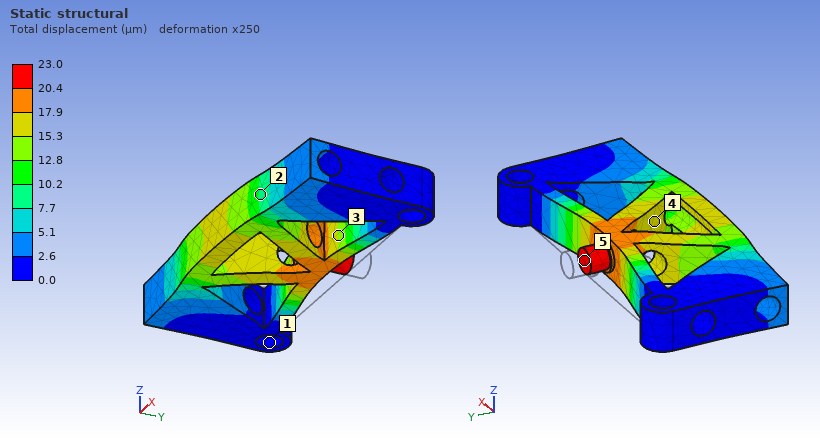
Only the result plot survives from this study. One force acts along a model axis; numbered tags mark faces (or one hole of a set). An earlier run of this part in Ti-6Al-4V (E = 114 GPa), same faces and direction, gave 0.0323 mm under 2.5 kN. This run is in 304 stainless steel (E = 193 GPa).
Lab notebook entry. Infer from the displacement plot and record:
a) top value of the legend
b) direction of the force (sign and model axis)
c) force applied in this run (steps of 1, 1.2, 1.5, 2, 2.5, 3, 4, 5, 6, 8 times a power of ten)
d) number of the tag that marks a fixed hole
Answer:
23.0 µm
-Y
3 kN
1
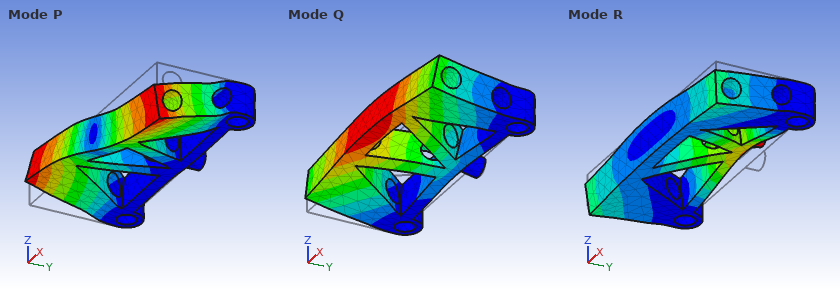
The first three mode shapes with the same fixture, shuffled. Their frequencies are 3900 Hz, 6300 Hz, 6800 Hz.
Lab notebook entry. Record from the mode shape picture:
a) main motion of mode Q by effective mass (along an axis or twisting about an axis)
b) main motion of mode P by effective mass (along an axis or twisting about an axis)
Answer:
along Z
twisting about Y
